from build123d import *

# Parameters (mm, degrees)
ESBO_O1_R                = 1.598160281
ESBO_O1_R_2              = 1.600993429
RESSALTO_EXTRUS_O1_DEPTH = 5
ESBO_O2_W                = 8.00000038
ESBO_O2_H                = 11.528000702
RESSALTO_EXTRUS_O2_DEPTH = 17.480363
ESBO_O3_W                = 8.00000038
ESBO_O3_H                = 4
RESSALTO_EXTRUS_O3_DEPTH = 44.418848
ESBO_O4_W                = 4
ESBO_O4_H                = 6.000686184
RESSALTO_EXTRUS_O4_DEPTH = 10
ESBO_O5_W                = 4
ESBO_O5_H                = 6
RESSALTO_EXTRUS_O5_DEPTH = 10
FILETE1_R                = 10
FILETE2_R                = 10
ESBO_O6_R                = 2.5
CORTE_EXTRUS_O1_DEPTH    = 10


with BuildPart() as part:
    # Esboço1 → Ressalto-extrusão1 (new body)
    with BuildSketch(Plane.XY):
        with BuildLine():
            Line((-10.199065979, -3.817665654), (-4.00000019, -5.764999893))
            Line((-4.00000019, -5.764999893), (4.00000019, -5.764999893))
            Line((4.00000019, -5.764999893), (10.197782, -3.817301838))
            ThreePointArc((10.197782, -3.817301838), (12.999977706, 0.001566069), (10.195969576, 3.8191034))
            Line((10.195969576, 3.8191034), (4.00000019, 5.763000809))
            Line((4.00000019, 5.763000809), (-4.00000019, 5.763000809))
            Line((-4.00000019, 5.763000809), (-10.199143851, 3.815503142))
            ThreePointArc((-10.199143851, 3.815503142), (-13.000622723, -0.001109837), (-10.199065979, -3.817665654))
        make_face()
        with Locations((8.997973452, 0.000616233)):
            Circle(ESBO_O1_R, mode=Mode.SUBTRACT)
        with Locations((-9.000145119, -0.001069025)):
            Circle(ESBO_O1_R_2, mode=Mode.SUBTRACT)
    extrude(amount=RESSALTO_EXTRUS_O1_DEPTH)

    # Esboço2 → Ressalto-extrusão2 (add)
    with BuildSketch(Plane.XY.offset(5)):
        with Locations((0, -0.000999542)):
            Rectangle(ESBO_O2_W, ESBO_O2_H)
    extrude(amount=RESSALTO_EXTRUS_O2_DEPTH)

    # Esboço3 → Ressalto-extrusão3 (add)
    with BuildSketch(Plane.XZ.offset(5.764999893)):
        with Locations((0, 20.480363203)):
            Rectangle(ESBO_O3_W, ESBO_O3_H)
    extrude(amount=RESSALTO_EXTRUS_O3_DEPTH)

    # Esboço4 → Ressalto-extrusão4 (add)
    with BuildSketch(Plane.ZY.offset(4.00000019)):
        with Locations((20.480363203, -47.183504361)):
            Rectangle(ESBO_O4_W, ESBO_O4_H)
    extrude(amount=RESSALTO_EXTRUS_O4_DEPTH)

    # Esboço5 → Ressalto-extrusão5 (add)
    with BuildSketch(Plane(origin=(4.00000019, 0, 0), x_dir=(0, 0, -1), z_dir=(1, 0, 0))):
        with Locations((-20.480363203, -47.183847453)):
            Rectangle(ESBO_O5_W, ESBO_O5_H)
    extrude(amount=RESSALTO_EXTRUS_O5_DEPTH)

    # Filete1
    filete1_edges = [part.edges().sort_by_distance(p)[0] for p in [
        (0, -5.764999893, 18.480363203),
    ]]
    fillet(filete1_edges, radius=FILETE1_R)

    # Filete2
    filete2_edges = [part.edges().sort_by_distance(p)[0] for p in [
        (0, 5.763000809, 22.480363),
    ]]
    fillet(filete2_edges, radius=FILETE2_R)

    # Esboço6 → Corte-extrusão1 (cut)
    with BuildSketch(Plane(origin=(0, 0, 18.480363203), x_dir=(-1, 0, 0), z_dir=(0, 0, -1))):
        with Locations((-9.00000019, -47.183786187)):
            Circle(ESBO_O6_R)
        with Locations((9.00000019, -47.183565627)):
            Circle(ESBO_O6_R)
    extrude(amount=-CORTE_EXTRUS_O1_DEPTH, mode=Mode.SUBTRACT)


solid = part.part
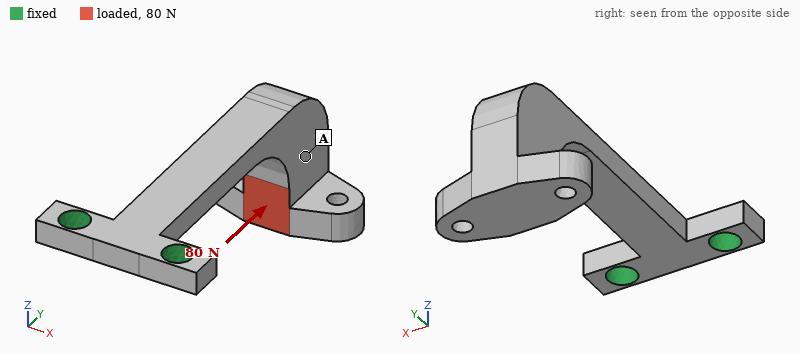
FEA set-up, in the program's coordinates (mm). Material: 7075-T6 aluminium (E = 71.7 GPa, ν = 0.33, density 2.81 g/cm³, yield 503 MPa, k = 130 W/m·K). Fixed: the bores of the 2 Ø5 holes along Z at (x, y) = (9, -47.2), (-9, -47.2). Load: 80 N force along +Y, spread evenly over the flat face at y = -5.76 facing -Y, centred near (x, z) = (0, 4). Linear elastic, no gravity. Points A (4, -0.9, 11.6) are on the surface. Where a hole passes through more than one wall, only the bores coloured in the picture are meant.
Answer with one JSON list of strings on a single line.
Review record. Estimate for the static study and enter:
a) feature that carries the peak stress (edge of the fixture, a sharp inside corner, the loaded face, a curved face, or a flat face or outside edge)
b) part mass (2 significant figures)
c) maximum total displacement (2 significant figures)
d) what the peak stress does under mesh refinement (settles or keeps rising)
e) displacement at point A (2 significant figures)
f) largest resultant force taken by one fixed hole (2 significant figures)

["a sharp inside corner", "13 g", "0.66 mm", "keeps rising", "0.49 mm", "42 N"]
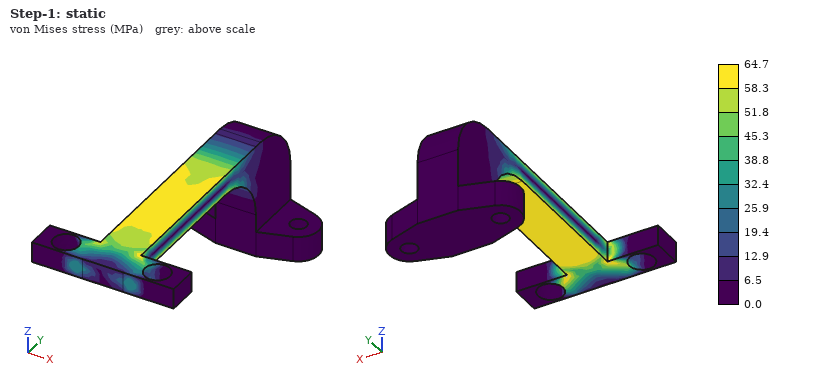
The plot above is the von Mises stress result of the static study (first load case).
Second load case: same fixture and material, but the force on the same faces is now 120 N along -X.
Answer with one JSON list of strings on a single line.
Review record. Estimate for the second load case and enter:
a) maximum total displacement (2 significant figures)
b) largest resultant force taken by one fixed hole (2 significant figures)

["0.78 mm", "440 N"]
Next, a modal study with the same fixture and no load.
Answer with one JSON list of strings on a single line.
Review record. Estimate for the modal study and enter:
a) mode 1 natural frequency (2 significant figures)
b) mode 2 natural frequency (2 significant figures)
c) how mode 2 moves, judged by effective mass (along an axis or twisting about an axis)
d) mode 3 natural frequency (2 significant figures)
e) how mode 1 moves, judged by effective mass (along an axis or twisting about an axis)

["470 Hz", "840 Hz", "along X", "2500 Hz", "along Z"]
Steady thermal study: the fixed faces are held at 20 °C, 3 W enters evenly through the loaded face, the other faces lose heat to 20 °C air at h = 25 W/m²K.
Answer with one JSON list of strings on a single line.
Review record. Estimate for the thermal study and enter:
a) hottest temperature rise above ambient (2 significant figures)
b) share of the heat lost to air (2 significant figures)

["24 K", "34 %"]
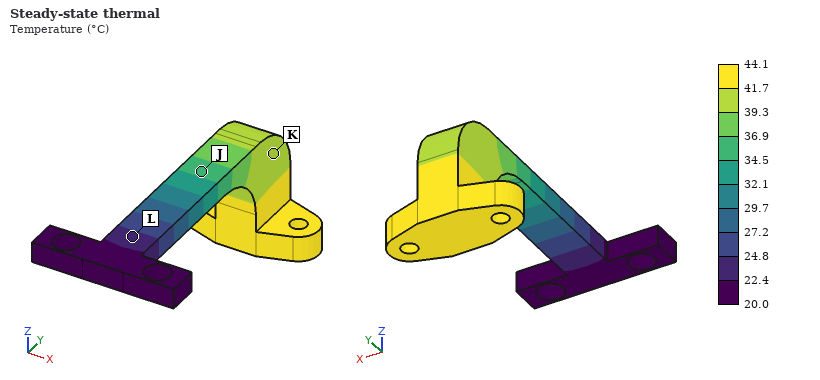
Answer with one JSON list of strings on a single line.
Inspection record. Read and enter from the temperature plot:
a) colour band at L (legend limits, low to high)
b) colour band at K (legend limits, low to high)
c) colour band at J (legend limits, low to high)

["22.4 to 24.8 °C", "39.3 to 41.7 °C", "34.5 to 36.9 °C"]
